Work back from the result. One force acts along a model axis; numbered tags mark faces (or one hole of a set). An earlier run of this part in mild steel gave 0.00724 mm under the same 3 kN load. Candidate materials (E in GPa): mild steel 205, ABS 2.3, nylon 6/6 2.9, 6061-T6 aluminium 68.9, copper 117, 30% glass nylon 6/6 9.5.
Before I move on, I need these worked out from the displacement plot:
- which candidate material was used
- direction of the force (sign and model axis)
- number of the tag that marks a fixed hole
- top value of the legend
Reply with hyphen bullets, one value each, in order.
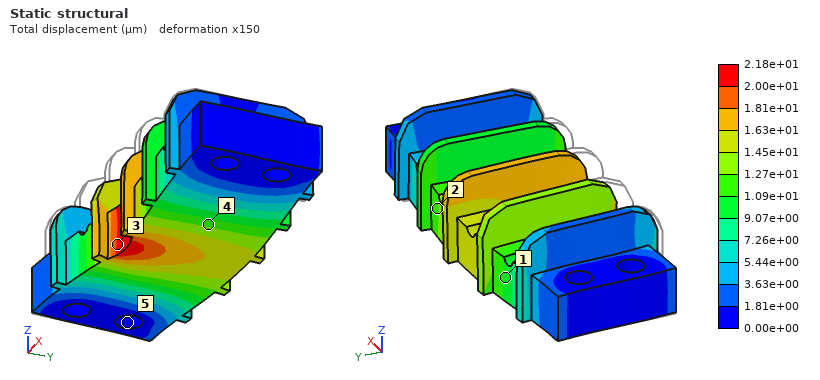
- 6061-T6 aluminium
- +Y
- 5
- 2.18e+01 µm
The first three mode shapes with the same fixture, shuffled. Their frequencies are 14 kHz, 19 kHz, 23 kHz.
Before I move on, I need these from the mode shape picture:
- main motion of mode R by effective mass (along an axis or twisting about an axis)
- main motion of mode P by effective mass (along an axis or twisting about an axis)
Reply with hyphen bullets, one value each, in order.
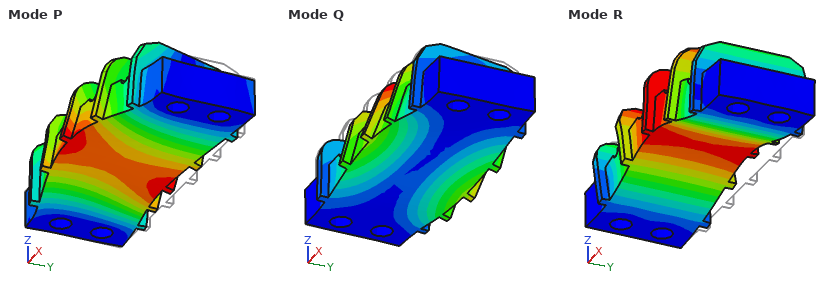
- along Z
- along Y
